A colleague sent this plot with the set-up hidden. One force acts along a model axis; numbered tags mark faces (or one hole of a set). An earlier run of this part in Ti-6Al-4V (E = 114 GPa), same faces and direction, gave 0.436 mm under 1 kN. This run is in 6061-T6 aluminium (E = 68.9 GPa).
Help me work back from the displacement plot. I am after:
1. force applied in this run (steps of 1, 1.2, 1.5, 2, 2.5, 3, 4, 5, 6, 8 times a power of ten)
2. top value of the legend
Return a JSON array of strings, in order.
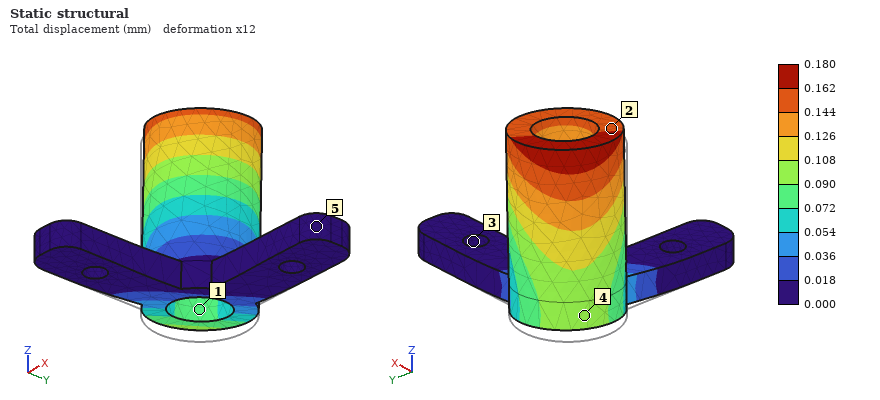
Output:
["250 N", "0.180 mm"]
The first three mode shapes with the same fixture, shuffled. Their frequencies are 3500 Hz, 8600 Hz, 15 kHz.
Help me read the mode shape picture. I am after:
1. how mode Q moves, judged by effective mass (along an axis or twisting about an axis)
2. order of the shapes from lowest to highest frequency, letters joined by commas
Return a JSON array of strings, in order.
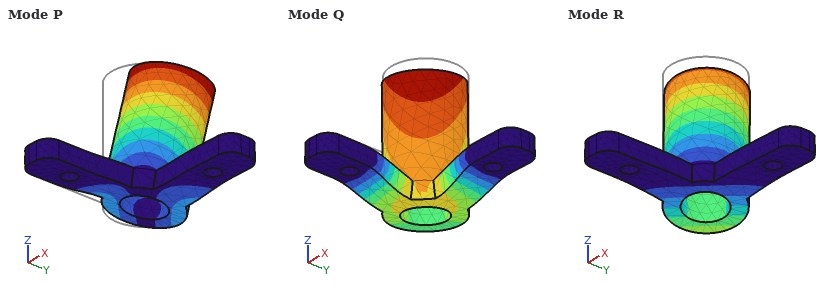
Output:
["along Z", "R, P, Q"]
